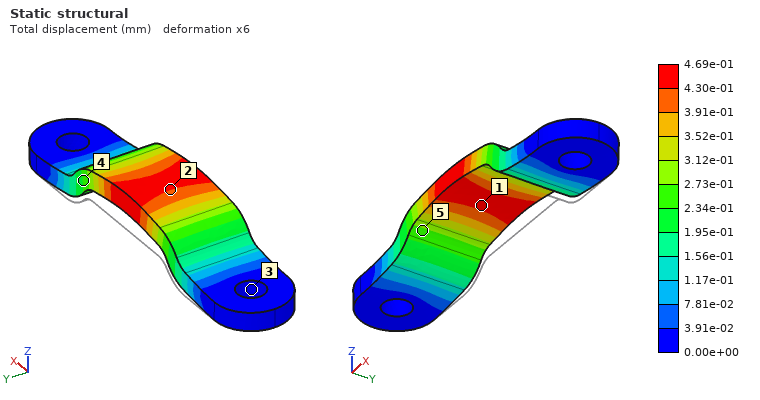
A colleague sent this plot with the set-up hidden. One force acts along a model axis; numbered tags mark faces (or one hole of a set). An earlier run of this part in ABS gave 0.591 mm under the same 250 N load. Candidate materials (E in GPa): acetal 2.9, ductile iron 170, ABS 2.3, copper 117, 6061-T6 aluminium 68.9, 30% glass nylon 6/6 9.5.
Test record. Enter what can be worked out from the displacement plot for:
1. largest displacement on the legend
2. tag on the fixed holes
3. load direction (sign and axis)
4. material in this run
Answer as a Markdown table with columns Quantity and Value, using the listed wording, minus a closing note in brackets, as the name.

| Quantity | Value |
|---|---|
| largest displacement on the legend | 4.69e-01 mm |
| tag on the fixed holes | 3 |
| load direction | +Z |
| material in this run | acetal |
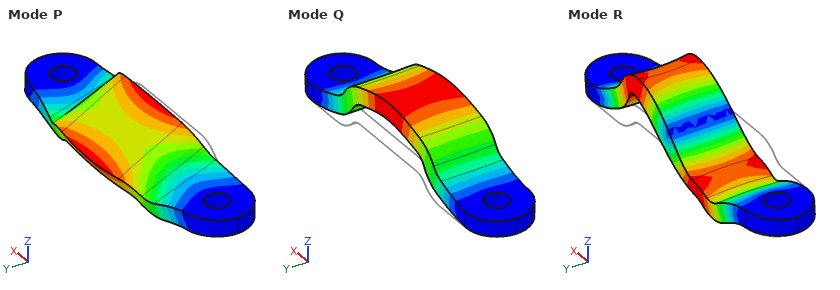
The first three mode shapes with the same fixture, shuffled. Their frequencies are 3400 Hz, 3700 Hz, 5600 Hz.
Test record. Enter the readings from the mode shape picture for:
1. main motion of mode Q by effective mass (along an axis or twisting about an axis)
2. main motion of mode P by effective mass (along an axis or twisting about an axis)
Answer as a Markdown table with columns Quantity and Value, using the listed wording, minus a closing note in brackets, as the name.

| Quantity | Value |
|---|---|
| main motion of mode Q by effective mass | along Z |
| main motion of mode P by effective mass | along Y |
